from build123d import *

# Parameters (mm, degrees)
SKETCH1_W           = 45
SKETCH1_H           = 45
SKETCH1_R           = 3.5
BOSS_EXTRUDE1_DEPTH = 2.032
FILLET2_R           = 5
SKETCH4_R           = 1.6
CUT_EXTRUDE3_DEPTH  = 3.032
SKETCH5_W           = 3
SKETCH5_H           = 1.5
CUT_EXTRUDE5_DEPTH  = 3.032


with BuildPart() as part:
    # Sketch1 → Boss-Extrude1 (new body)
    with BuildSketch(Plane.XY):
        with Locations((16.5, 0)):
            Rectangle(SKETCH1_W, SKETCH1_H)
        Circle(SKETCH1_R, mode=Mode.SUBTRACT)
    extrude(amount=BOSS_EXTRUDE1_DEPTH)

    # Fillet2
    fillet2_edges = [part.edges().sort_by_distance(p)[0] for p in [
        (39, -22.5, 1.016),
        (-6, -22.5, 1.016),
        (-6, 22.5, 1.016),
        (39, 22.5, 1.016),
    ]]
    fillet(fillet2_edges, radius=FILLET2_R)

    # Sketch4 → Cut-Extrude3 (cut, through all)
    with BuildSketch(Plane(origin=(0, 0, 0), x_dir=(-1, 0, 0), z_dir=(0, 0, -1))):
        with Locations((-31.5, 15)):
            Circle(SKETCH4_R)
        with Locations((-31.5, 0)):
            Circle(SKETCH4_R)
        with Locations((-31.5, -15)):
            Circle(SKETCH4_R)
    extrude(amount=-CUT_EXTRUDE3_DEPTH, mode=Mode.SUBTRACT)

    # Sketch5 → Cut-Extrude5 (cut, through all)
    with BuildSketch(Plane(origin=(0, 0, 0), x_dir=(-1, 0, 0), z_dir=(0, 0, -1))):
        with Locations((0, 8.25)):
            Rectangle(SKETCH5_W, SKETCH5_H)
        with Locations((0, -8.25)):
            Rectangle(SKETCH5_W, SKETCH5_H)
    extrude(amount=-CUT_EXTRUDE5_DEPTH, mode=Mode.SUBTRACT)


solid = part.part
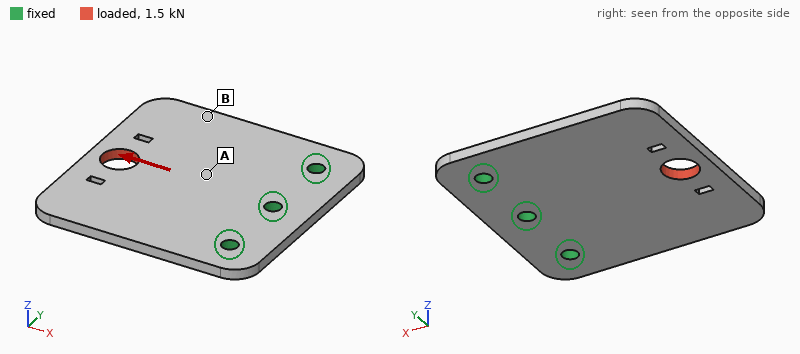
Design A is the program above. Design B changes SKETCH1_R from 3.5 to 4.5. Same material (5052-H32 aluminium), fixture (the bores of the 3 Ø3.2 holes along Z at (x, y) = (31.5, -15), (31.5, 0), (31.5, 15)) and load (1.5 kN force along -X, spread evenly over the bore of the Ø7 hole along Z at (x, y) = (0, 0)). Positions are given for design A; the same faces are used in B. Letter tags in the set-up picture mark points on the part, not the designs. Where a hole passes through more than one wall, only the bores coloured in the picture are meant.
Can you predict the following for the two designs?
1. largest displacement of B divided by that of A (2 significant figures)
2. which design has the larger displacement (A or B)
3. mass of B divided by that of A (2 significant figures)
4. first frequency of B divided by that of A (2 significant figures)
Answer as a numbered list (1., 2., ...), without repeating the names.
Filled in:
1. 1.3
2. B
3. 0.99
4. 1.0
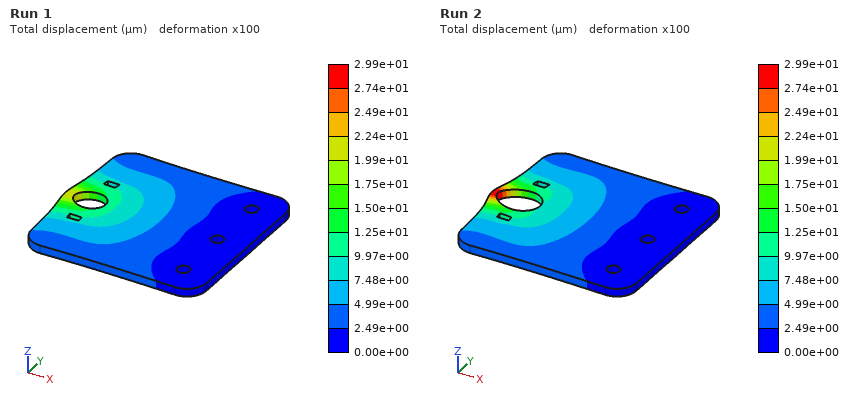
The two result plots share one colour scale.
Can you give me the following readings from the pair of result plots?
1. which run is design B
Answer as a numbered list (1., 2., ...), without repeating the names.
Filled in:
1. Run 2
